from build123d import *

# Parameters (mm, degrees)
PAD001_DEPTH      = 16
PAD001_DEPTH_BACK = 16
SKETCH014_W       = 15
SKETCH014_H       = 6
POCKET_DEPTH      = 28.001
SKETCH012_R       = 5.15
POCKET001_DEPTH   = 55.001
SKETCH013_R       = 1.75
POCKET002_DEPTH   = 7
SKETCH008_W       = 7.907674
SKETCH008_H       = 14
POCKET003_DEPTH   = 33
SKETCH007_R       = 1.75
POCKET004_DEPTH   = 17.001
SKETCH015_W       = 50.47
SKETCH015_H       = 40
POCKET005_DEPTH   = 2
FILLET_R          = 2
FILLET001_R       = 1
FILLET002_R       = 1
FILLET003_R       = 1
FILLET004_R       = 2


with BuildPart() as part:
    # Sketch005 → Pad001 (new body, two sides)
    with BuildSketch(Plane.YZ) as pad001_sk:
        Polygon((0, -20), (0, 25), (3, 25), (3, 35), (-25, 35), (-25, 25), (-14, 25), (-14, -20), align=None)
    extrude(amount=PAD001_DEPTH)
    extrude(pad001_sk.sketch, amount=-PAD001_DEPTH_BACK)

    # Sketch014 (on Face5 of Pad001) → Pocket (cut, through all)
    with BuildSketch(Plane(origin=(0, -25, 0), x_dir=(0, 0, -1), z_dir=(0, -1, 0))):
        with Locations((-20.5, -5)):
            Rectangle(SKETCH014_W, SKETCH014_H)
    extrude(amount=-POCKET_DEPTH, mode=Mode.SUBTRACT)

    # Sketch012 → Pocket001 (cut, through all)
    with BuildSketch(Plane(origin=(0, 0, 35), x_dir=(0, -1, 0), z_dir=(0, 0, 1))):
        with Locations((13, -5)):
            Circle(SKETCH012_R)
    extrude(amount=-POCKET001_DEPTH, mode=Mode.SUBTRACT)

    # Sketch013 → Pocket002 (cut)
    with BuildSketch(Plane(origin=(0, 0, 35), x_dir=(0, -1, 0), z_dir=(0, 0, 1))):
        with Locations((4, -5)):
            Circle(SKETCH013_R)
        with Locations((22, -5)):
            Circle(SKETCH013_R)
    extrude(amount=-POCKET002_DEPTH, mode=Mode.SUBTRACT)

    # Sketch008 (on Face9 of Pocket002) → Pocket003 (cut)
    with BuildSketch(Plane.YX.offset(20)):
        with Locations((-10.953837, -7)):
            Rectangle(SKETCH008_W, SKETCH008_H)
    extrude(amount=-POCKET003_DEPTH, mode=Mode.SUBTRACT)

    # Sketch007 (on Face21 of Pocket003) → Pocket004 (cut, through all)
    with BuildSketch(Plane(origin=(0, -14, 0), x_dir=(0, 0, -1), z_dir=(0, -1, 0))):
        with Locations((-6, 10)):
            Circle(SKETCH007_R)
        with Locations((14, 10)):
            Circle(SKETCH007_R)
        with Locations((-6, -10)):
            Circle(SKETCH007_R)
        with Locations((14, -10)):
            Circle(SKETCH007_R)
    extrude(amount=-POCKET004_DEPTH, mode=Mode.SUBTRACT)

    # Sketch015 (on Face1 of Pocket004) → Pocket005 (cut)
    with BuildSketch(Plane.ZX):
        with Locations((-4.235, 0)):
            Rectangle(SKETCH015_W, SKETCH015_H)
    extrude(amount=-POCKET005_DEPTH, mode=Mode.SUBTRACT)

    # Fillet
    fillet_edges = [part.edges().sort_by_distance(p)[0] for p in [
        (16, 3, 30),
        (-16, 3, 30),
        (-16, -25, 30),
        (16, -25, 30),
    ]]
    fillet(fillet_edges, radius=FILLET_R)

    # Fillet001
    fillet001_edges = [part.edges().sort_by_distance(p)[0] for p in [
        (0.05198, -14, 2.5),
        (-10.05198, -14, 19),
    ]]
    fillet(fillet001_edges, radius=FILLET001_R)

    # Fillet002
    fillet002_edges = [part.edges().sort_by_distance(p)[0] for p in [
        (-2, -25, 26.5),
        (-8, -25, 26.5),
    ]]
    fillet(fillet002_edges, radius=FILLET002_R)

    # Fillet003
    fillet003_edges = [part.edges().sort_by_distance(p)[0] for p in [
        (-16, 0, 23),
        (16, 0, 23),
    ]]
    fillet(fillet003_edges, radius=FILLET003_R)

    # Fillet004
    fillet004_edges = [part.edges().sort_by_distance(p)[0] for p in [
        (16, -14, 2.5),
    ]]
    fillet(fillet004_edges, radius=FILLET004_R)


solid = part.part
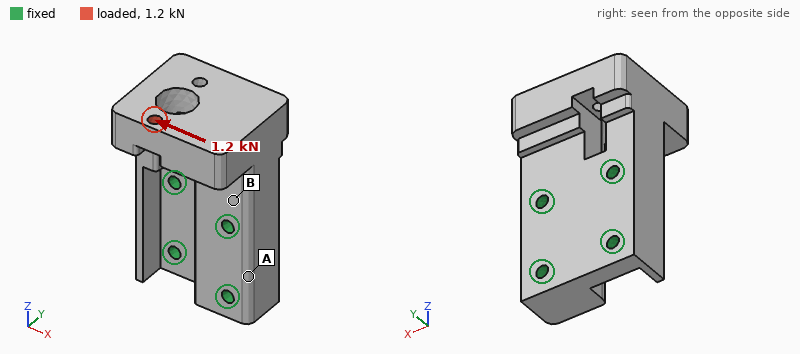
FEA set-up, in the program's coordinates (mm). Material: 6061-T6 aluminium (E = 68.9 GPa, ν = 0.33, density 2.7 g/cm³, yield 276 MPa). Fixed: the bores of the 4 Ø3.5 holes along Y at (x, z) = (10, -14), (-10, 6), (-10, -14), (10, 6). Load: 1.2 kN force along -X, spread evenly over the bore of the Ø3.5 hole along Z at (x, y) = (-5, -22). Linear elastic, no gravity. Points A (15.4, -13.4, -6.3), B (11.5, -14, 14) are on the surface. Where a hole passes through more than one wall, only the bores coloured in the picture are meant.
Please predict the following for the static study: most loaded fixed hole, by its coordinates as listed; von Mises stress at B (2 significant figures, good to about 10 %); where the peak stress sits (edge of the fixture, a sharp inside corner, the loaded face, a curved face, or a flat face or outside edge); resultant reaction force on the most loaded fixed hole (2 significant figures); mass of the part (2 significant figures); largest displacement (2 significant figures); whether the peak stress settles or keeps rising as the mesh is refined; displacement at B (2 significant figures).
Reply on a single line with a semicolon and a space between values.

(10, 6); 32 MPa; edge of the fixture; 1.7 kN; 55 g; 52 µm; keeps rising; 8.0 µm
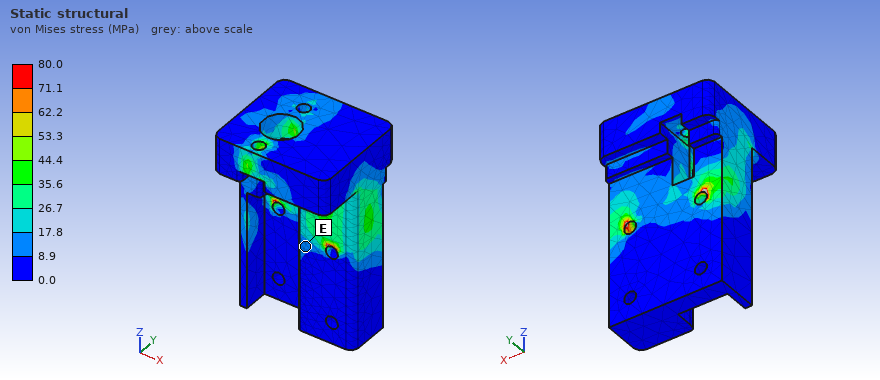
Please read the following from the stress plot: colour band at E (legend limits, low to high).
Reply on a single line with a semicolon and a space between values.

8.9 to 17.8 MPa
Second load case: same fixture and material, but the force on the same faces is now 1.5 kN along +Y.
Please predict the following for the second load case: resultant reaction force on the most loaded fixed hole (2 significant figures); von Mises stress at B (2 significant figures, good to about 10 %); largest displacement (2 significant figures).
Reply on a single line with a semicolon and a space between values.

1.1 kN; 57 MPa; 0.11 mm
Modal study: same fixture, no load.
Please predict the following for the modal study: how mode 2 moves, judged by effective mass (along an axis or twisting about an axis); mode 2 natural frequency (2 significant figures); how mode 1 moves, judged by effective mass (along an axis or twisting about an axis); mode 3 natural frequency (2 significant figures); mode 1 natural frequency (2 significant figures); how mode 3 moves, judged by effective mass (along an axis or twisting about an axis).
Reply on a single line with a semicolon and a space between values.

along X; 8100 Hz; along Y; 11 kHz; 5200 Hz; along X
